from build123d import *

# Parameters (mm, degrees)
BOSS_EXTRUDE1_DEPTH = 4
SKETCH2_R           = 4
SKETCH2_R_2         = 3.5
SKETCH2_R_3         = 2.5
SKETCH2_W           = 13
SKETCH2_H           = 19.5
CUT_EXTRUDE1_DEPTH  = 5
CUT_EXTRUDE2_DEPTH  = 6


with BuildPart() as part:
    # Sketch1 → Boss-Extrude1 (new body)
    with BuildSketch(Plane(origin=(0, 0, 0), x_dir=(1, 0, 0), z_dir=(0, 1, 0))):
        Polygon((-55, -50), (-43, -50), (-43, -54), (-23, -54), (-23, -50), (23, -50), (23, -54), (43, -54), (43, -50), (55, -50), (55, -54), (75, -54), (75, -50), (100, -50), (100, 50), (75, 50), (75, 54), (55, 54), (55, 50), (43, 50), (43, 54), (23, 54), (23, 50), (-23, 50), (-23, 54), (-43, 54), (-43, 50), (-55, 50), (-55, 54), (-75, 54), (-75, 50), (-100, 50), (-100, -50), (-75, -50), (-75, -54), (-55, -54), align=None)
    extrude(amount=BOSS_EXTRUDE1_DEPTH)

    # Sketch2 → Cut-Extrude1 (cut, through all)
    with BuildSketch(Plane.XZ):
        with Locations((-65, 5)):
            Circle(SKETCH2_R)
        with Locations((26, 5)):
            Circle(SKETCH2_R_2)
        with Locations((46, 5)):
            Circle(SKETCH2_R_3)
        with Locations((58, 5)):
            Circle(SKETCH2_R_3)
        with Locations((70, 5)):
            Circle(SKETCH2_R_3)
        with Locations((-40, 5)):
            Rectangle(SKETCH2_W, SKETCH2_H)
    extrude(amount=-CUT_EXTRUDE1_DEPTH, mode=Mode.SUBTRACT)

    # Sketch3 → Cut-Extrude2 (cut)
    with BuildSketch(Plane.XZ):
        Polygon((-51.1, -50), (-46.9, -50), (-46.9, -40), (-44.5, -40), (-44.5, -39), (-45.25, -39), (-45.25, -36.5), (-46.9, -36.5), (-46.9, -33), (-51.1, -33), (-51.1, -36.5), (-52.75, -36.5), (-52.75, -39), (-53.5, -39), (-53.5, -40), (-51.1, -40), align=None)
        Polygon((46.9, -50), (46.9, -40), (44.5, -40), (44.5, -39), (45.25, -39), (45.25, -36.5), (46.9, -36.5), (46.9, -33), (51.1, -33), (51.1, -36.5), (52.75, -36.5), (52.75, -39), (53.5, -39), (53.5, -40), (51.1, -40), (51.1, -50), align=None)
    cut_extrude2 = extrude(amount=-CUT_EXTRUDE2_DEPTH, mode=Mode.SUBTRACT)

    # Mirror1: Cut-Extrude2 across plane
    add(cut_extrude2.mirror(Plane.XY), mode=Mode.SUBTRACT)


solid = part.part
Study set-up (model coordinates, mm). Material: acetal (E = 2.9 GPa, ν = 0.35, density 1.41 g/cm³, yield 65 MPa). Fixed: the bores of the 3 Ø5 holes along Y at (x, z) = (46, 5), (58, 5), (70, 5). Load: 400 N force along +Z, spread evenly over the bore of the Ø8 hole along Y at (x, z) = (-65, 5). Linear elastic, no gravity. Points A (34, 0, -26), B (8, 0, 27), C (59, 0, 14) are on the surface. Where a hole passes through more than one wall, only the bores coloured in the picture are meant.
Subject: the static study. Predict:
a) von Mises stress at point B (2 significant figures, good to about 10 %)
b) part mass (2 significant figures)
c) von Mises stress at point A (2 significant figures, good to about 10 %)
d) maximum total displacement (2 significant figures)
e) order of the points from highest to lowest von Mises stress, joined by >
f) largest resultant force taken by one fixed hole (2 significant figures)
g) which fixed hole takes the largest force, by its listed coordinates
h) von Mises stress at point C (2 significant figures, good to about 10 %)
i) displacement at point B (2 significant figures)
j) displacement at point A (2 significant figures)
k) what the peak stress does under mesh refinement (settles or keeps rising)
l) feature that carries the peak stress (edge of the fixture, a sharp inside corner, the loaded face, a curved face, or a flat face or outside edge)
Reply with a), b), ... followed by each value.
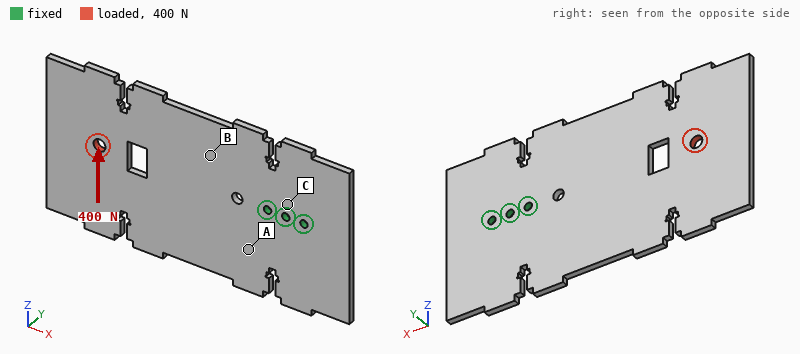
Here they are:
a) 3.1 MPa
b) 110 g
c) 7.6 MPa
d) 2.5 mm
e) C > A > B
f) 2.0 kN
g) (46, 5)
h) 15 MPa
i) 0.69 mm
j) 0.45 mm
k) keeps rising
l) edge of the fixture
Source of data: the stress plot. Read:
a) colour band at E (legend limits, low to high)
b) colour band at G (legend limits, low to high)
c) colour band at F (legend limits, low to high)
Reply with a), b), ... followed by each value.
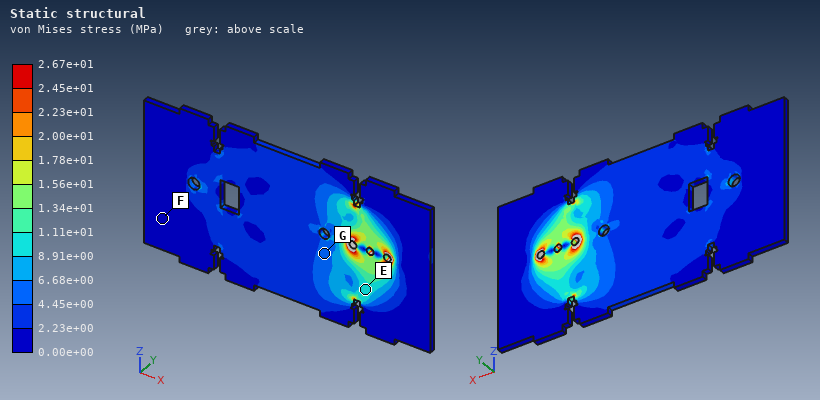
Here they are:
a) 8.91e+00 to 1.11e+01 MPa
b) 4.45e+00 to 6.68e+00 MPa
c) 0.00e+00 to 2.23e+00 MPa
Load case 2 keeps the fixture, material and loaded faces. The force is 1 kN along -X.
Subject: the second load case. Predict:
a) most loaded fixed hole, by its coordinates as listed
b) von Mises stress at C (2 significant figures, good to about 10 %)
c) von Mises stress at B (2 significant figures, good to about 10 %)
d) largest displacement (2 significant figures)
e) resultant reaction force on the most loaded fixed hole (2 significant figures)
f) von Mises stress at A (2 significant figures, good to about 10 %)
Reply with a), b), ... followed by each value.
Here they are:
a) (46, 5)
b) 3.5 MPa
c) 3.6 MPa
d) 0.24 mm
e) 510 N
f) 1.9 MPa
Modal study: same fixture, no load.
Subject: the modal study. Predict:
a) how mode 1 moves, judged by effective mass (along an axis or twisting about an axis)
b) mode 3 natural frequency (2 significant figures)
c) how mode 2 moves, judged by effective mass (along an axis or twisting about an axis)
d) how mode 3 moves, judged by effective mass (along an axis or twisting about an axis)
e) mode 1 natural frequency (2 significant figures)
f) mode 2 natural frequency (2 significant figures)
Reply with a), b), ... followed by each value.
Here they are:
a) along Y
b) 210 Hz
c) twisting about X
d) along Y
e) 39 Hz
f) 100 Hz
